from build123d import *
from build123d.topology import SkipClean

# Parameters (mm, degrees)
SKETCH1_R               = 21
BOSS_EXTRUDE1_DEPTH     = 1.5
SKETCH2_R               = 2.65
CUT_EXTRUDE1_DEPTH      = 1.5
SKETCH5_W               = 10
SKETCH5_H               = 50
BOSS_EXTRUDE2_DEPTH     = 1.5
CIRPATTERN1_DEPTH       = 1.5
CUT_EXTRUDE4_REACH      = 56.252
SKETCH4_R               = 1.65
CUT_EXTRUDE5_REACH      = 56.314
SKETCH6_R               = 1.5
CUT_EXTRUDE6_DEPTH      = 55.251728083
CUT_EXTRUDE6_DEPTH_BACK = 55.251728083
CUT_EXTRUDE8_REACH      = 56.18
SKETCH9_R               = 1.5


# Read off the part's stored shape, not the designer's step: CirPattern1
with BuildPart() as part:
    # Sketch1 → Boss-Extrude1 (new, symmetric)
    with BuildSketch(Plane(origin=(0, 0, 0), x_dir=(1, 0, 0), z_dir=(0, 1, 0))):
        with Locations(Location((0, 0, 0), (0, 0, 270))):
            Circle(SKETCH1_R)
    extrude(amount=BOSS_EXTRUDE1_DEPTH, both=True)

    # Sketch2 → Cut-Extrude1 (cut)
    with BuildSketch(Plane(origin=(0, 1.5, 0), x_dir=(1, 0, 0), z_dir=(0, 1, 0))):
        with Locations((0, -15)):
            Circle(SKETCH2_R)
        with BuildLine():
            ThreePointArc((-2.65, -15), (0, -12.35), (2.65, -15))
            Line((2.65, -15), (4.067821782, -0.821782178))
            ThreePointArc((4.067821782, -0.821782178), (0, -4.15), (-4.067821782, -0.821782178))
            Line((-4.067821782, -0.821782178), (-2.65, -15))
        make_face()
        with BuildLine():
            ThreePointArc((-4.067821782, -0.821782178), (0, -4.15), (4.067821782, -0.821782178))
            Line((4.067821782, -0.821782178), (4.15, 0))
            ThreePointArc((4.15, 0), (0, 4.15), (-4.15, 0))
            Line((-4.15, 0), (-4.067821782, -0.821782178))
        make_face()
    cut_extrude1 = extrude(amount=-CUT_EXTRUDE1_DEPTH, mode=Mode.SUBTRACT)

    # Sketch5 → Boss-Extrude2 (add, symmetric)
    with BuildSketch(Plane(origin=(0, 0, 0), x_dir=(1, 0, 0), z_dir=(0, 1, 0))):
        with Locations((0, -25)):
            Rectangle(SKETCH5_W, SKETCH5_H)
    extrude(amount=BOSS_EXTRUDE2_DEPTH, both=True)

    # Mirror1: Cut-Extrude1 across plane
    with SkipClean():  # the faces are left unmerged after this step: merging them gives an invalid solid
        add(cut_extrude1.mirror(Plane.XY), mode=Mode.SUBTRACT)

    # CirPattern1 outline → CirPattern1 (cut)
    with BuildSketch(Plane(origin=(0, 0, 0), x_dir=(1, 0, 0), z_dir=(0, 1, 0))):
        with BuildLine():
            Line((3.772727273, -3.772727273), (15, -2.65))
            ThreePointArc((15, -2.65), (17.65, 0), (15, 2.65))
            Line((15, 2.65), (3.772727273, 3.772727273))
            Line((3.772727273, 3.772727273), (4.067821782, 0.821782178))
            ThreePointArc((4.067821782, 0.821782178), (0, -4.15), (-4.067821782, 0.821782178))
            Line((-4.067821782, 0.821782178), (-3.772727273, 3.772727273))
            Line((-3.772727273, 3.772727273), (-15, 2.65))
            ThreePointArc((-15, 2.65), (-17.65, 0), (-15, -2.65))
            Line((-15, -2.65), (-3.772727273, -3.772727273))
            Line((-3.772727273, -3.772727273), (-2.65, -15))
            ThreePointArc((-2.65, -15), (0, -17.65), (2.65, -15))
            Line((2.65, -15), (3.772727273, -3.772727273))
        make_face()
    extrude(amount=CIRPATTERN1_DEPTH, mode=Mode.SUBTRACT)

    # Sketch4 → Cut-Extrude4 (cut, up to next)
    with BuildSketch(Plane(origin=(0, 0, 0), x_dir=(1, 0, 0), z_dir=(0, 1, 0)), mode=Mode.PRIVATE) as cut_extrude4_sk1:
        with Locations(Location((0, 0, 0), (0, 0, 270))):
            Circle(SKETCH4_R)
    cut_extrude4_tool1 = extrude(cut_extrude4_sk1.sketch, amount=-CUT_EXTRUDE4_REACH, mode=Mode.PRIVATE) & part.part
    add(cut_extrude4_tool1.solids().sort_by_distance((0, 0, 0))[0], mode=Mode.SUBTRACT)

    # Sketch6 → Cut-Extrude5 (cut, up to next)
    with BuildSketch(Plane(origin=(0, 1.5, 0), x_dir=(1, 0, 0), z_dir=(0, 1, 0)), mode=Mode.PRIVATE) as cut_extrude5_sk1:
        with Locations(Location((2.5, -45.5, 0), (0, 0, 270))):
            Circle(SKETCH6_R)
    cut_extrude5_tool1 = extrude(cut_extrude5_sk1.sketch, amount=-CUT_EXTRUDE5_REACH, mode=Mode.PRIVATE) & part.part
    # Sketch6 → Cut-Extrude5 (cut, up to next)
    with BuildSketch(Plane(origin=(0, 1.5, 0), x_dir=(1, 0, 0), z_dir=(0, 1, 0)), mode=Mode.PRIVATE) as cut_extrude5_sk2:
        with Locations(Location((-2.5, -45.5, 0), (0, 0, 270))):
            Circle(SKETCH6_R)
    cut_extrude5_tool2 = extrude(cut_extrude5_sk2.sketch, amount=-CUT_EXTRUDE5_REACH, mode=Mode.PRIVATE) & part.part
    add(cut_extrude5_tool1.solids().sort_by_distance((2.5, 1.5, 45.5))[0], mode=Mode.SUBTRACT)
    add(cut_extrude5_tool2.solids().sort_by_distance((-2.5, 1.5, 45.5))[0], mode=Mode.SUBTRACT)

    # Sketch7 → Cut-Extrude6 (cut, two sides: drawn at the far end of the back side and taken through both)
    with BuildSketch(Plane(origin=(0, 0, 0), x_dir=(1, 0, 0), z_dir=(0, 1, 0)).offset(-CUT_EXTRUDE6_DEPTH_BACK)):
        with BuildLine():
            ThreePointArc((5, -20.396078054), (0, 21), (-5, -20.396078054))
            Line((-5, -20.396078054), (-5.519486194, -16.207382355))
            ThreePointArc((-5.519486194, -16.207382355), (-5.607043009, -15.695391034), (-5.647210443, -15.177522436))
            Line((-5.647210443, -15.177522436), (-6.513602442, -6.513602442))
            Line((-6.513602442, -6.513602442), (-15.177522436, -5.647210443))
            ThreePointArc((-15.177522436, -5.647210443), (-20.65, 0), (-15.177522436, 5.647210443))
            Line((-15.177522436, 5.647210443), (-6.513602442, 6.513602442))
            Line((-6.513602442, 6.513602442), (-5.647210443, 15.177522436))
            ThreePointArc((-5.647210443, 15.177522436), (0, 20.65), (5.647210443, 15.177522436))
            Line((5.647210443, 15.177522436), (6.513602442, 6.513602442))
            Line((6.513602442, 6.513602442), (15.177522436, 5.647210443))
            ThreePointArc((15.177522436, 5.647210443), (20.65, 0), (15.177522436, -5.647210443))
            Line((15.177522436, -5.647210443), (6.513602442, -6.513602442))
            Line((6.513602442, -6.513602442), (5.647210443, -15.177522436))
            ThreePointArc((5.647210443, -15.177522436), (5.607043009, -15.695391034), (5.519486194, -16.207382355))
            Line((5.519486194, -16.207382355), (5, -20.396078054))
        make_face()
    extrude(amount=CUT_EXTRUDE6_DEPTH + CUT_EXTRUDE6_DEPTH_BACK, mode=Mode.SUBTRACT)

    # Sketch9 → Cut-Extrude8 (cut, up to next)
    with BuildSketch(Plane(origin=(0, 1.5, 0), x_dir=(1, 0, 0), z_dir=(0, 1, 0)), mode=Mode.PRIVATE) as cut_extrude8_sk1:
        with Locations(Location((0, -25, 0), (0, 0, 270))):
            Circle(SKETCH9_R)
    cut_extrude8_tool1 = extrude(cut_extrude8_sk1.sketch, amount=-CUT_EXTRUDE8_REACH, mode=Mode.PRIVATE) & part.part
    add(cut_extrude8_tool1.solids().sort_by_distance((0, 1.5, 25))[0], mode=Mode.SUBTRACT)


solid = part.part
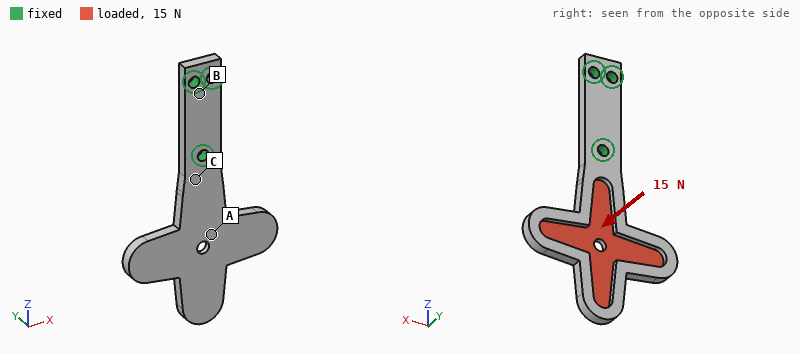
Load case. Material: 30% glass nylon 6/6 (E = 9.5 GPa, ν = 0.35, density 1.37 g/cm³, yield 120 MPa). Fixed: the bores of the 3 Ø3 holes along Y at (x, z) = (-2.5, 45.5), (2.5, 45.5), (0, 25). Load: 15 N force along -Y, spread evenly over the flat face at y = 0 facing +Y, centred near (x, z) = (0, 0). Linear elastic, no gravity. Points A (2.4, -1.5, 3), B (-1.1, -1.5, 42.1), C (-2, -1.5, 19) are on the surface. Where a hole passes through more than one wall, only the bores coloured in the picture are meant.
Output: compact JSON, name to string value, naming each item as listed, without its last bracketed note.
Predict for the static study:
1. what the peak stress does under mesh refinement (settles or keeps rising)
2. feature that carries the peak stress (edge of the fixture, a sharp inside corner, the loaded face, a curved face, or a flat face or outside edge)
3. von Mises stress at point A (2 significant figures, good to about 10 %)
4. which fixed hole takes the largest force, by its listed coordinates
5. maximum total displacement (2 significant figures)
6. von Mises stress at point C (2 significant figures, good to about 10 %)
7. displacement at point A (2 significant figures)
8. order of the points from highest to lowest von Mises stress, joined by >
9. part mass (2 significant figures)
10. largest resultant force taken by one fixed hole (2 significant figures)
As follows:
{"what the peak stress does under mesh refinement": "keeps rising", "feature that carries the peak stress": "edge of the fixture", "von Mises stress at point A": "6.4 MPa", "which fixed hole takes the largest force, by its listed coordinates": "(0, 25)", "maximum total displacement": "0.96 mm", "von Mises stress at point C": "18 MPa", "displacement at point A": "0.31 mm", "order of the points from highest to lowest von Mises stress, joined by >": "C > A > B", "part mass": "3.6 g", "largest resultant force taken by one fixed hole": "16 N"}
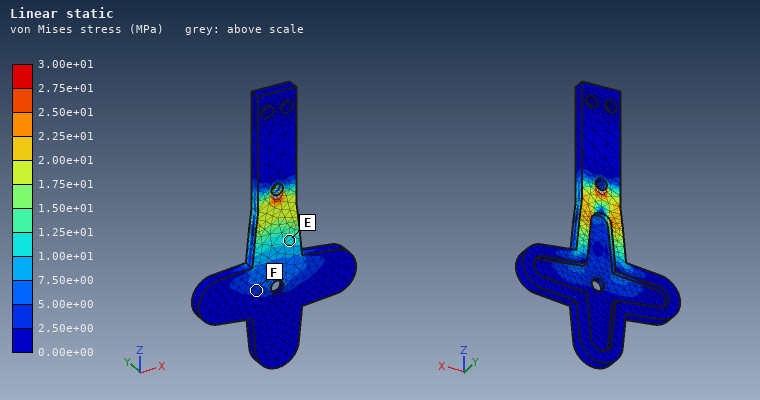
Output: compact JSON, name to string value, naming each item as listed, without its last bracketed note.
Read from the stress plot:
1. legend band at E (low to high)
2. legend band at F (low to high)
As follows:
{"legend band at E": "1.00e+01 to 1.25e+01 MPa", "legend band at F": "2.50e+00 to 5.00e+00 MPa"}
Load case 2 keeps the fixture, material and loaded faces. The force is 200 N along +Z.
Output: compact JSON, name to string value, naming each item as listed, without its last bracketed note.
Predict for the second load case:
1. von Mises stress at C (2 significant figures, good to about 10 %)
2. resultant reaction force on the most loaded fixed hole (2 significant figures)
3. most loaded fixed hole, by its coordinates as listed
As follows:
{"von Mises stress at C": "6.5 MPa", "resultant reaction force on the most loaded fixed hole": "190 N", "most loaded fixed hole, by its coordinates as listed": "(0, 25)"}
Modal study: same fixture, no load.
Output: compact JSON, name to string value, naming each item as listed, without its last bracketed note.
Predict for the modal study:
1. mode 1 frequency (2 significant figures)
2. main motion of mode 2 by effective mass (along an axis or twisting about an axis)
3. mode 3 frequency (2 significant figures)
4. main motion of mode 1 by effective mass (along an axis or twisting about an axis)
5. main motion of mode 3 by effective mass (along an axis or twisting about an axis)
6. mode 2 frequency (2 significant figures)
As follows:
{"mode 1 frequency": "530 Hz", "main motion of mode 2 by effective mass": "twisting about Z", "mode 3 frequency": "1500 Hz", "main motion of mode 1 by effective mass": "along Y", "main motion of mode 3 by effective mass": "along X", "mode 2 frequency": "970 Hz"}
